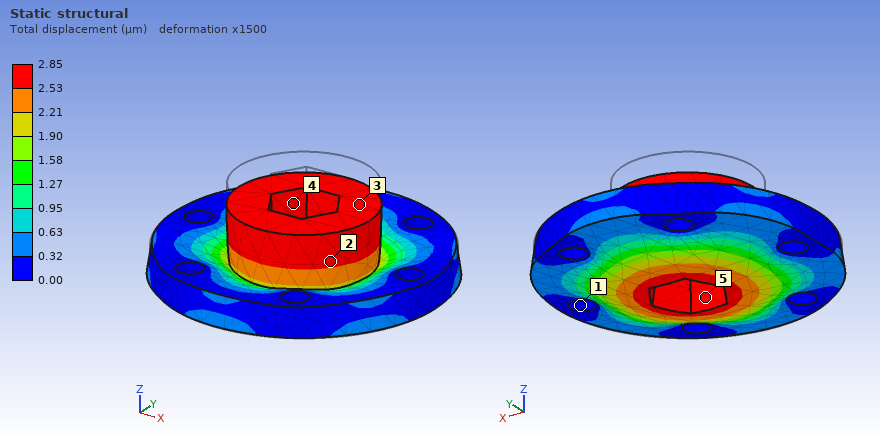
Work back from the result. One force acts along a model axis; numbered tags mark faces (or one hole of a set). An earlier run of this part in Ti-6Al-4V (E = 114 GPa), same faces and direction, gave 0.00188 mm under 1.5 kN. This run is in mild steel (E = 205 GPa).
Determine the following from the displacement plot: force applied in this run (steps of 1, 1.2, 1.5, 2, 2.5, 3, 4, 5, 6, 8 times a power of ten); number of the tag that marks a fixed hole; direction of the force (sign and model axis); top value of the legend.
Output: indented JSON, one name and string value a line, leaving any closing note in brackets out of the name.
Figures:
{
  "force applied in this run": "4 kN",
  "number of the tag that marks a fixed hole": "1",
  "direction of the force": "-Z",
  "top value of the legend": "2.85 µm"
}
